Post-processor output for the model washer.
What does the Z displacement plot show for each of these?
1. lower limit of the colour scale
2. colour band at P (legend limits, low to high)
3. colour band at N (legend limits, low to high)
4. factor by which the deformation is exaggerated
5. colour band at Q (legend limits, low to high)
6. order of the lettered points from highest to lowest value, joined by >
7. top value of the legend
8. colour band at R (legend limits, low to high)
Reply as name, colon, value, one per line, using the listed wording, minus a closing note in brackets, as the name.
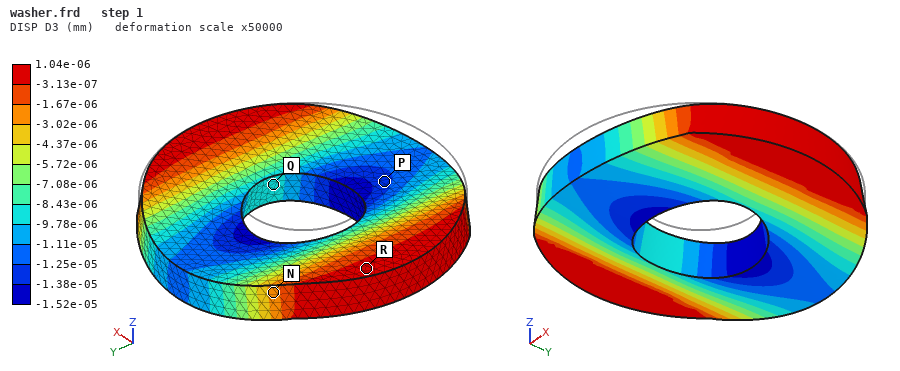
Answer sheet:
lower limit of the colour scale: -1.52e-05 mm
colour band at P: -1.38e-05 to -1.25e-05 mm
colour band at N: -3.02e-06 to -1.67e-06 mm
factor by which the deformation is exaggerated: 50000
colour band at Q: -9.78e-06 to -8.43e-06 mm
order of the lettered points from highest to lowest value, joined by >: R > N > Q > P
top value of the legend: 1.04e-06 mm
colour band at R: -3.13e-07 to 1.04e-06 mm
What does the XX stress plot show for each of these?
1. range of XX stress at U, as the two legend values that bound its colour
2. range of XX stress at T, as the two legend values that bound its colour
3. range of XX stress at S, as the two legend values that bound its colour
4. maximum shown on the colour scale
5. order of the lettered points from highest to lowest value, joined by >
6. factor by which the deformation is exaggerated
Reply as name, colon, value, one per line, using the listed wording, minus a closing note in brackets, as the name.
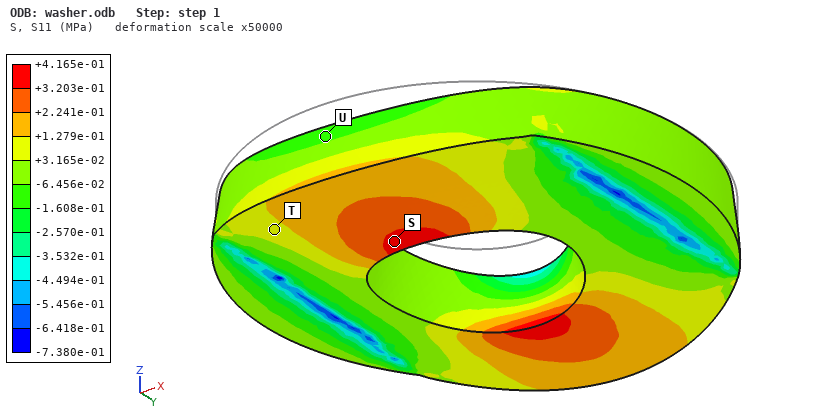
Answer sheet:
range of XX stress at U, as the two legend values that bound its colour: -1.608e-01 to -6.456e-02 MPa
range of XX stress at T, as the two legend values that bound its colour: +3.165e-02 to +1.279e-01 MPa
range of XX stress at S, as the two legend values that bound its colour: +3.203e-01 to +4.165e-01 MPa
maximum shown on the colour scale: +4.165e-01 MPa
order of the lettered points from highest to lowest value, joined by >: S > T > U
factor by which the deformation is exaggerated: 50000
